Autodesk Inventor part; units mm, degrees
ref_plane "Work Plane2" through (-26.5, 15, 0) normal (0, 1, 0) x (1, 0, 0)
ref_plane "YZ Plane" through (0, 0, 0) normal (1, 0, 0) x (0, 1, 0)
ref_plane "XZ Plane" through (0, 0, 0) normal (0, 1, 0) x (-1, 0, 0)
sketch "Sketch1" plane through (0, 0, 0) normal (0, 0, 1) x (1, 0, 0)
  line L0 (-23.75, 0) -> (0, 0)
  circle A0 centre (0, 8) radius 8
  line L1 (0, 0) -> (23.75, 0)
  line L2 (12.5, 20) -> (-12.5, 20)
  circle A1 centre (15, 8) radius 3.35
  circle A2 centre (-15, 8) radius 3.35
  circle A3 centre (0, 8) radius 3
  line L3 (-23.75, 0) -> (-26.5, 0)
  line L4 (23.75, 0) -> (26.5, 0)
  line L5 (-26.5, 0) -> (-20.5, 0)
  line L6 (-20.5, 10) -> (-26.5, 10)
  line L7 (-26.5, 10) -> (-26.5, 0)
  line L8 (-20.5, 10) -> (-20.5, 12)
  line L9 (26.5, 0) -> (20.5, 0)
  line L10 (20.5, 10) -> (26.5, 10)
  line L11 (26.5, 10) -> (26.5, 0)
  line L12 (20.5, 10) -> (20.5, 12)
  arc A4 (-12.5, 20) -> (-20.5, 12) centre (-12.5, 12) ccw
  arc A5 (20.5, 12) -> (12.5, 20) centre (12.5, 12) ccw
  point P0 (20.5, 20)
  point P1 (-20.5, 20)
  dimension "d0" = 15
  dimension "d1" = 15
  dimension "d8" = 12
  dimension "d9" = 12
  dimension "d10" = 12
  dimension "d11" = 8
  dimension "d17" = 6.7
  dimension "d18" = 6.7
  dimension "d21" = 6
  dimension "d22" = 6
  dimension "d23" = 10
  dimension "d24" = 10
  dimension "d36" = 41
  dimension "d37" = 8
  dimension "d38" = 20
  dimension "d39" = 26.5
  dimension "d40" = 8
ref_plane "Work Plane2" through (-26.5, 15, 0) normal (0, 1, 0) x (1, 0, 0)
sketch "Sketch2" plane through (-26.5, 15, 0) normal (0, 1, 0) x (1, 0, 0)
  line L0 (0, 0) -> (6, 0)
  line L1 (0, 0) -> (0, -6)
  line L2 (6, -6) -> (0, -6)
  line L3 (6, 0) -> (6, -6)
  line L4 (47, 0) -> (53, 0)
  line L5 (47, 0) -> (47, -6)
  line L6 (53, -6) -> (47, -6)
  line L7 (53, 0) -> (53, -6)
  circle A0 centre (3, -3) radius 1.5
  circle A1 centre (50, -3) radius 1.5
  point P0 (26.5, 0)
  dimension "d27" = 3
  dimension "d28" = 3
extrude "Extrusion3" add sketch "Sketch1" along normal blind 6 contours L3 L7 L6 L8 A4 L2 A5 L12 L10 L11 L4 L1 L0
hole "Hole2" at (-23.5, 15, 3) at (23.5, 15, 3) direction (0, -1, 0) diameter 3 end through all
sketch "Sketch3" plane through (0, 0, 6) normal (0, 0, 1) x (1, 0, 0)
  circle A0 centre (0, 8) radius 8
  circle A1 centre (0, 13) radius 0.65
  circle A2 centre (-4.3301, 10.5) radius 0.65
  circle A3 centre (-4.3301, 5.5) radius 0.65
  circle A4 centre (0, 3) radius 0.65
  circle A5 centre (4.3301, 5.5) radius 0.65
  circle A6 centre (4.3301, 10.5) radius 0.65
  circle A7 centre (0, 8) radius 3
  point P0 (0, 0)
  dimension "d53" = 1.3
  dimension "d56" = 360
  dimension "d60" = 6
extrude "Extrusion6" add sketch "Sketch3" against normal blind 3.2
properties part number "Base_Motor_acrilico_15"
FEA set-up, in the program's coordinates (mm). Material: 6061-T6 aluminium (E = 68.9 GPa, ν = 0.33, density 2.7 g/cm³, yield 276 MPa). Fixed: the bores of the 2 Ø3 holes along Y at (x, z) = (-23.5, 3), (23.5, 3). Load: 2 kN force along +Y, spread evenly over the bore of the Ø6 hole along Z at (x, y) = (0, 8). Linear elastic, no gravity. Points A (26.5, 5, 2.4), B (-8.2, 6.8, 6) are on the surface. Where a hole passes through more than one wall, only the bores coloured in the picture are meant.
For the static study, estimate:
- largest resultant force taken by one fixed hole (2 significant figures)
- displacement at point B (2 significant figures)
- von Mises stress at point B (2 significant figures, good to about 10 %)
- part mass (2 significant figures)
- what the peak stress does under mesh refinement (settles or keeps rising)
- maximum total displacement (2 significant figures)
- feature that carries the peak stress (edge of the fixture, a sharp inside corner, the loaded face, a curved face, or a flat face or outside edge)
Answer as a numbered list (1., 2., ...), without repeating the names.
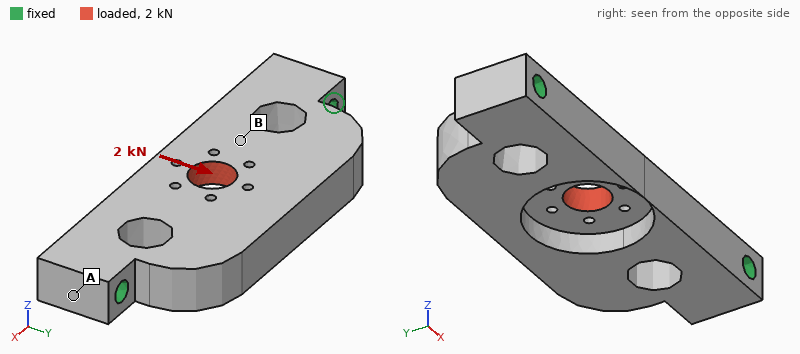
1. 1.2 kN
2. 22 µm
3. 45 MPa
4. 11 g
5. keeps rising
6. 33 µm
7. a sharp inside corner
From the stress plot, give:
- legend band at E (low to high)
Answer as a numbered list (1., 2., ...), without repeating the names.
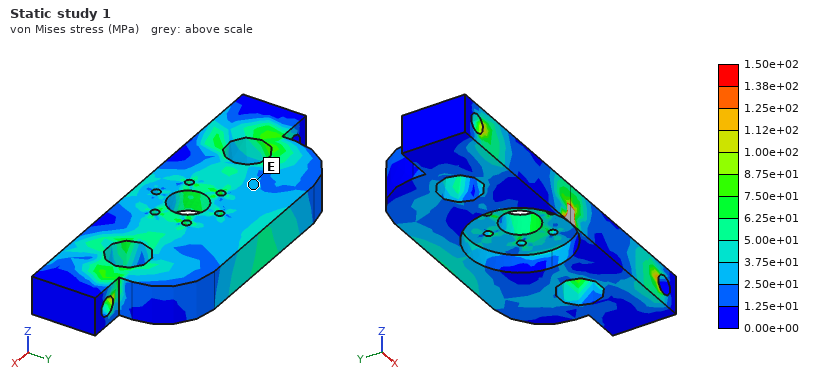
1. 2.50e+01 to 3.75e+01 MPa
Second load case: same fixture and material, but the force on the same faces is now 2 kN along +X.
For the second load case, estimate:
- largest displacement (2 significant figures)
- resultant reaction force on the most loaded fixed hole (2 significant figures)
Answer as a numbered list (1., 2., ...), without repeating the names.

1. 10 µm
2. 1.0 kN
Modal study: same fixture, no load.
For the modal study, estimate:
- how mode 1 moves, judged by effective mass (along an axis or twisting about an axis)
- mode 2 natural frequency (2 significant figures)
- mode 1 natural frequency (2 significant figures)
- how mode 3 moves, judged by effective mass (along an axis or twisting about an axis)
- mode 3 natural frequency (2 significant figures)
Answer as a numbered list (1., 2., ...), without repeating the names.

1. along Z
2. 15 kHz
3. 8000 Hz
4. twisting about Y
5. 19 kHz
